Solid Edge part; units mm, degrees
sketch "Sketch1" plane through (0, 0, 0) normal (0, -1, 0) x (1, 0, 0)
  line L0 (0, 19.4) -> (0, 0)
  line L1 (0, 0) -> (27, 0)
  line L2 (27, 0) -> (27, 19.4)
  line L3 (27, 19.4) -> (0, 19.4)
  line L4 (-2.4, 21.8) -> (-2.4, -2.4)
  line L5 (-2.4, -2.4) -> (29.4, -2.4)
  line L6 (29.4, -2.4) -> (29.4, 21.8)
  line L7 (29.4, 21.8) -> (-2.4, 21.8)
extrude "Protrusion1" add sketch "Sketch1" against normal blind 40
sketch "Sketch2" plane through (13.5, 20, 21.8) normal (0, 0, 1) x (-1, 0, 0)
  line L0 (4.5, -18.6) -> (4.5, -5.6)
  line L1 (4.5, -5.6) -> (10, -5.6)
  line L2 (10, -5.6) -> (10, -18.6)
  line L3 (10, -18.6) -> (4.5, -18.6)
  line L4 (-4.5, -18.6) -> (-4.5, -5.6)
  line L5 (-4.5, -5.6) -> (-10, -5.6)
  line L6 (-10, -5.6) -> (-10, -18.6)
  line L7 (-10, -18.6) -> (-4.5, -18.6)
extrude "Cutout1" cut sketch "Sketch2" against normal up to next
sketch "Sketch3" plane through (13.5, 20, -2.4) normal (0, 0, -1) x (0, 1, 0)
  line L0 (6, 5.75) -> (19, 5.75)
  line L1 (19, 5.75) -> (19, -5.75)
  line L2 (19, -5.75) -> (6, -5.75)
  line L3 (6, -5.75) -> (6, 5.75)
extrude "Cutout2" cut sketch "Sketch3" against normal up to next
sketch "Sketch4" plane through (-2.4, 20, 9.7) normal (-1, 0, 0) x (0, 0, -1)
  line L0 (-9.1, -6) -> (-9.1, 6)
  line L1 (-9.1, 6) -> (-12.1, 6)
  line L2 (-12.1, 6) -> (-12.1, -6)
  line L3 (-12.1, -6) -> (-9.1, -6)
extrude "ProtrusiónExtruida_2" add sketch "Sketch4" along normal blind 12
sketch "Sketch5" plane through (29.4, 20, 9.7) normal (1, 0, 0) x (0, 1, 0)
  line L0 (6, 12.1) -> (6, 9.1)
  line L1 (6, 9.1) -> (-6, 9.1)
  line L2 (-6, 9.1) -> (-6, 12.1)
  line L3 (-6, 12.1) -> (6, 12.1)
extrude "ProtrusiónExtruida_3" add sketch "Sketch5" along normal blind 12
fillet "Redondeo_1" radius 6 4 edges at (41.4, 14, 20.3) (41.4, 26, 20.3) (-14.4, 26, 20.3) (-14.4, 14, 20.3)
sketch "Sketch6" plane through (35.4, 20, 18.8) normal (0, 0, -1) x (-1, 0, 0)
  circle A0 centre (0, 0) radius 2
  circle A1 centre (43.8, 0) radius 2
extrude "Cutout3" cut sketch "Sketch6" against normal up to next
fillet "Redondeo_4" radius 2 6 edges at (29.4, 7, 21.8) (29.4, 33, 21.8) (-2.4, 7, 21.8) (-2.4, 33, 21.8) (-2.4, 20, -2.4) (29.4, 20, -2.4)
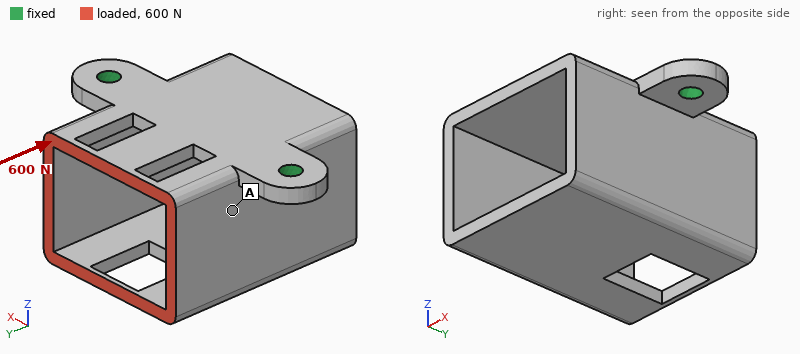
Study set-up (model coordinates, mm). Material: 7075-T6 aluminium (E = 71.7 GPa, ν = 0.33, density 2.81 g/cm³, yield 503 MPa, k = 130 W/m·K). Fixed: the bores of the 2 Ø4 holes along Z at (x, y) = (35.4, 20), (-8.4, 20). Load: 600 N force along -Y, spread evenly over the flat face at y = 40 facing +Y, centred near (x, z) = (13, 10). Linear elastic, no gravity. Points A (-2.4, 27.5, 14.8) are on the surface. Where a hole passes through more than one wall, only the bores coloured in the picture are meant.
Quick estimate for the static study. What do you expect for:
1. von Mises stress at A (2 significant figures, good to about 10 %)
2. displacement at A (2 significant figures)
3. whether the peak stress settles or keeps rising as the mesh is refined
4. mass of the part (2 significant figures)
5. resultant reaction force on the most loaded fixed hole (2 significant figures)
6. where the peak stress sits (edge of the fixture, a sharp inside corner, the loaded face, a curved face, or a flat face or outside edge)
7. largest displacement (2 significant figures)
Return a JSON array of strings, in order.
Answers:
["16 MPa", "0.052 mm", "keeps rising", "27 g", "300 N", "edge of the fixture", "0.19 mm"]
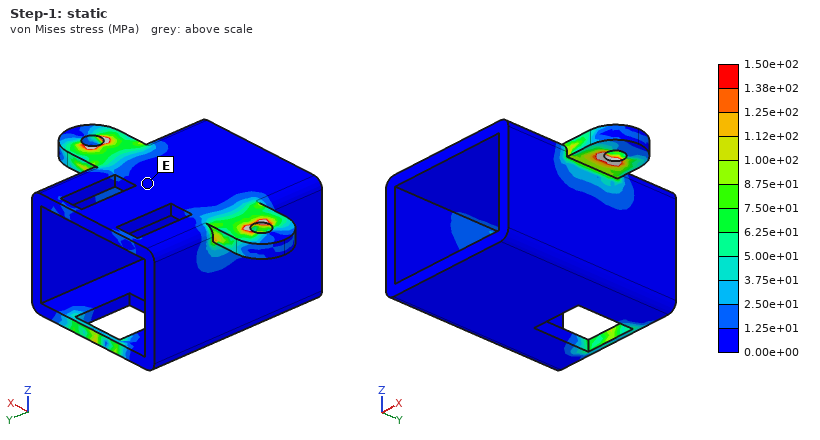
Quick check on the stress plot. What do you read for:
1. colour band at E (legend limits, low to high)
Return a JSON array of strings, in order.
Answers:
["0.00e+00 to 1.25e+01 MPa"]
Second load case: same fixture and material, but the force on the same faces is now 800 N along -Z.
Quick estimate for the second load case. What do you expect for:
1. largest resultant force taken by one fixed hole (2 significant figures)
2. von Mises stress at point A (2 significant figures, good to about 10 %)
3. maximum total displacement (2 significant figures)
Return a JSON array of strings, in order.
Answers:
["400 N", "67 MPa", "0.48 mm"]
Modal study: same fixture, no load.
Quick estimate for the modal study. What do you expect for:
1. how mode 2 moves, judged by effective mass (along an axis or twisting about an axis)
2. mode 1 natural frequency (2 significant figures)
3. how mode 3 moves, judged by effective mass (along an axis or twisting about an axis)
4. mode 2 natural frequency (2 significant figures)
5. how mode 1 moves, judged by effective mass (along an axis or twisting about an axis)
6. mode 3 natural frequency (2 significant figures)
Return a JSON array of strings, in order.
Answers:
["along X", "1900 Hz", "twisting about Z", "3100 Hz", "along Y", "4400 Hz"]
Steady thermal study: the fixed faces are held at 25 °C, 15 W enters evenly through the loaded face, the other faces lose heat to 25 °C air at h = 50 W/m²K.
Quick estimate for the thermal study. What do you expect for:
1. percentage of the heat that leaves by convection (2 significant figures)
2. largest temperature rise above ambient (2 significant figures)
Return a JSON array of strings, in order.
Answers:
["32 %", "33 K"]
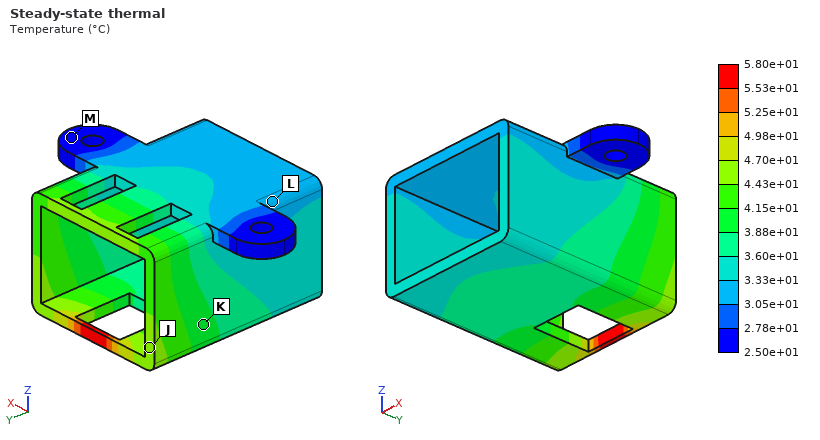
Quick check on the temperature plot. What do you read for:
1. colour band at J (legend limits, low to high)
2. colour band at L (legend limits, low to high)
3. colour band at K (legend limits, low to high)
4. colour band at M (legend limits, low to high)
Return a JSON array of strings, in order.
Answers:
["4.43e+01 to 4.70e+01 °C", "3.05e+01 to 3.33e+01 °C", "3.88e+01 to 4.15e+01 °C", "2.50e+01 to 2.78e+01 °C"]
